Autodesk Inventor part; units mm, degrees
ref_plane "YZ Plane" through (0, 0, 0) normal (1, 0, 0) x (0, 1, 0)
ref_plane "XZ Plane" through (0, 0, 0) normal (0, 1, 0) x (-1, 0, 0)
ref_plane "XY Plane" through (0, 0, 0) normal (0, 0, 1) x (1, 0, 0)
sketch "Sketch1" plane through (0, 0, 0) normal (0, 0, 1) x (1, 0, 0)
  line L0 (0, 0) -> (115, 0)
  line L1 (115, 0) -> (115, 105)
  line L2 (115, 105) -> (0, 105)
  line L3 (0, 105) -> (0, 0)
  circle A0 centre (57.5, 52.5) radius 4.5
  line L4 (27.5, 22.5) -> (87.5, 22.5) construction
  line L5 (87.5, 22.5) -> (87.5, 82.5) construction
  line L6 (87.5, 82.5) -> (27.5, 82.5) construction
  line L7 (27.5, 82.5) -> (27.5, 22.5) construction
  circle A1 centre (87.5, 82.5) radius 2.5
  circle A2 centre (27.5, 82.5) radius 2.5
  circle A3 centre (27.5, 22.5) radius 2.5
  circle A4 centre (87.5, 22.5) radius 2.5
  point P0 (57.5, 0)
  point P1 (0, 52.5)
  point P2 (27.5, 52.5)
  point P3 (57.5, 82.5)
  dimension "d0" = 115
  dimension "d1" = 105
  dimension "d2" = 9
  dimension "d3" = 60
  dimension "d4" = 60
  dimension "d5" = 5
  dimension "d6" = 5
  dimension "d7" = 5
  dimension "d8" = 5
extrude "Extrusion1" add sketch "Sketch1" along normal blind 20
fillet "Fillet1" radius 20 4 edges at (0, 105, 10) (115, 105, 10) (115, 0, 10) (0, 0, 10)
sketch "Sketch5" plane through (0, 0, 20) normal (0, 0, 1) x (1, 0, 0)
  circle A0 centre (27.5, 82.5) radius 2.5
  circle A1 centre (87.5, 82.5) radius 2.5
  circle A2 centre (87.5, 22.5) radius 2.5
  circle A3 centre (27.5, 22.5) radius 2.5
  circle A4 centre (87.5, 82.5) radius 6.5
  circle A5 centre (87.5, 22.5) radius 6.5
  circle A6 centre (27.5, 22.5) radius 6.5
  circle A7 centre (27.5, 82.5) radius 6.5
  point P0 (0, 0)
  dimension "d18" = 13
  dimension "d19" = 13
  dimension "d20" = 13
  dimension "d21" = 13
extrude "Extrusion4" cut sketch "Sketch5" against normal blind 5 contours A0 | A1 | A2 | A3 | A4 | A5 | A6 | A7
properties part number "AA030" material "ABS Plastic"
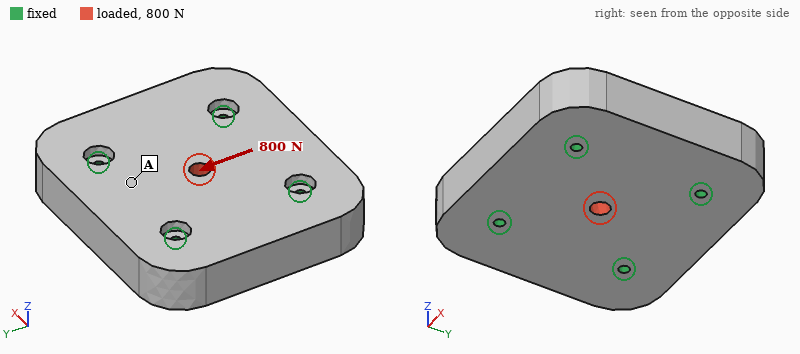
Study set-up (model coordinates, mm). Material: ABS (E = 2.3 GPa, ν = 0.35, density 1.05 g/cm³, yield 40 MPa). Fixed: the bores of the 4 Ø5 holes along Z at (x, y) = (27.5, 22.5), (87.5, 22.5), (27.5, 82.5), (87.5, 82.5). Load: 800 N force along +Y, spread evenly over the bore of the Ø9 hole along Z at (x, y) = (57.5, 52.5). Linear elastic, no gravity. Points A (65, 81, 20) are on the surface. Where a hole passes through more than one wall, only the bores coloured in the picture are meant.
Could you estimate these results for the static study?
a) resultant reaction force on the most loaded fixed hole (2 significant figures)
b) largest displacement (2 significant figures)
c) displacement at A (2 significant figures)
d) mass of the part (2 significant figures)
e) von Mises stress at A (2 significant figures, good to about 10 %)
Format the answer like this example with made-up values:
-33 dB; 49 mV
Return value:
210 N; 15 µm; 7.4 µm; 240 g; 0.27 MPa
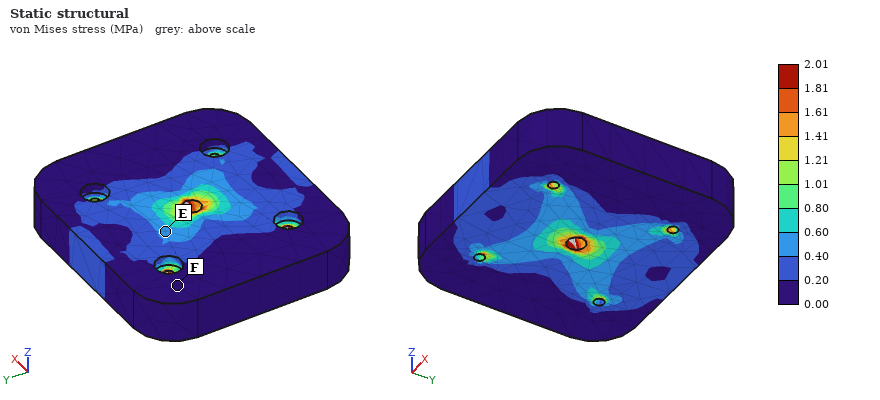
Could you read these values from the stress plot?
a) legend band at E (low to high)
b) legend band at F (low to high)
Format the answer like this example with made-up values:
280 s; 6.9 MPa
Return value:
0.40 to 0.60 MPa; 0.00 to 0.20 MPa
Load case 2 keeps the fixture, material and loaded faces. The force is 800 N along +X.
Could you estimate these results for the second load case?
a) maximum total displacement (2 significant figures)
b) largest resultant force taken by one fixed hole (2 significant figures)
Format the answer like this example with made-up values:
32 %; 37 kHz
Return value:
15 µm; 210 N
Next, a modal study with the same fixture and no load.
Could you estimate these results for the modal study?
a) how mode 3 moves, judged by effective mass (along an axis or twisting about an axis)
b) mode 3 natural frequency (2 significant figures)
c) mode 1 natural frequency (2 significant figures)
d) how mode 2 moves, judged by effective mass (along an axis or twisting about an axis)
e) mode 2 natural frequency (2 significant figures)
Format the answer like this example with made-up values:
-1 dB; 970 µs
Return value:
along Z; 3400 Hz; 2700 Hz; twisting about Y; 2900 Hz
